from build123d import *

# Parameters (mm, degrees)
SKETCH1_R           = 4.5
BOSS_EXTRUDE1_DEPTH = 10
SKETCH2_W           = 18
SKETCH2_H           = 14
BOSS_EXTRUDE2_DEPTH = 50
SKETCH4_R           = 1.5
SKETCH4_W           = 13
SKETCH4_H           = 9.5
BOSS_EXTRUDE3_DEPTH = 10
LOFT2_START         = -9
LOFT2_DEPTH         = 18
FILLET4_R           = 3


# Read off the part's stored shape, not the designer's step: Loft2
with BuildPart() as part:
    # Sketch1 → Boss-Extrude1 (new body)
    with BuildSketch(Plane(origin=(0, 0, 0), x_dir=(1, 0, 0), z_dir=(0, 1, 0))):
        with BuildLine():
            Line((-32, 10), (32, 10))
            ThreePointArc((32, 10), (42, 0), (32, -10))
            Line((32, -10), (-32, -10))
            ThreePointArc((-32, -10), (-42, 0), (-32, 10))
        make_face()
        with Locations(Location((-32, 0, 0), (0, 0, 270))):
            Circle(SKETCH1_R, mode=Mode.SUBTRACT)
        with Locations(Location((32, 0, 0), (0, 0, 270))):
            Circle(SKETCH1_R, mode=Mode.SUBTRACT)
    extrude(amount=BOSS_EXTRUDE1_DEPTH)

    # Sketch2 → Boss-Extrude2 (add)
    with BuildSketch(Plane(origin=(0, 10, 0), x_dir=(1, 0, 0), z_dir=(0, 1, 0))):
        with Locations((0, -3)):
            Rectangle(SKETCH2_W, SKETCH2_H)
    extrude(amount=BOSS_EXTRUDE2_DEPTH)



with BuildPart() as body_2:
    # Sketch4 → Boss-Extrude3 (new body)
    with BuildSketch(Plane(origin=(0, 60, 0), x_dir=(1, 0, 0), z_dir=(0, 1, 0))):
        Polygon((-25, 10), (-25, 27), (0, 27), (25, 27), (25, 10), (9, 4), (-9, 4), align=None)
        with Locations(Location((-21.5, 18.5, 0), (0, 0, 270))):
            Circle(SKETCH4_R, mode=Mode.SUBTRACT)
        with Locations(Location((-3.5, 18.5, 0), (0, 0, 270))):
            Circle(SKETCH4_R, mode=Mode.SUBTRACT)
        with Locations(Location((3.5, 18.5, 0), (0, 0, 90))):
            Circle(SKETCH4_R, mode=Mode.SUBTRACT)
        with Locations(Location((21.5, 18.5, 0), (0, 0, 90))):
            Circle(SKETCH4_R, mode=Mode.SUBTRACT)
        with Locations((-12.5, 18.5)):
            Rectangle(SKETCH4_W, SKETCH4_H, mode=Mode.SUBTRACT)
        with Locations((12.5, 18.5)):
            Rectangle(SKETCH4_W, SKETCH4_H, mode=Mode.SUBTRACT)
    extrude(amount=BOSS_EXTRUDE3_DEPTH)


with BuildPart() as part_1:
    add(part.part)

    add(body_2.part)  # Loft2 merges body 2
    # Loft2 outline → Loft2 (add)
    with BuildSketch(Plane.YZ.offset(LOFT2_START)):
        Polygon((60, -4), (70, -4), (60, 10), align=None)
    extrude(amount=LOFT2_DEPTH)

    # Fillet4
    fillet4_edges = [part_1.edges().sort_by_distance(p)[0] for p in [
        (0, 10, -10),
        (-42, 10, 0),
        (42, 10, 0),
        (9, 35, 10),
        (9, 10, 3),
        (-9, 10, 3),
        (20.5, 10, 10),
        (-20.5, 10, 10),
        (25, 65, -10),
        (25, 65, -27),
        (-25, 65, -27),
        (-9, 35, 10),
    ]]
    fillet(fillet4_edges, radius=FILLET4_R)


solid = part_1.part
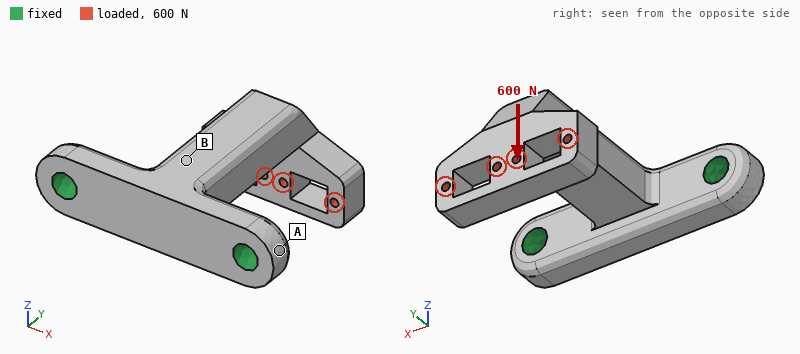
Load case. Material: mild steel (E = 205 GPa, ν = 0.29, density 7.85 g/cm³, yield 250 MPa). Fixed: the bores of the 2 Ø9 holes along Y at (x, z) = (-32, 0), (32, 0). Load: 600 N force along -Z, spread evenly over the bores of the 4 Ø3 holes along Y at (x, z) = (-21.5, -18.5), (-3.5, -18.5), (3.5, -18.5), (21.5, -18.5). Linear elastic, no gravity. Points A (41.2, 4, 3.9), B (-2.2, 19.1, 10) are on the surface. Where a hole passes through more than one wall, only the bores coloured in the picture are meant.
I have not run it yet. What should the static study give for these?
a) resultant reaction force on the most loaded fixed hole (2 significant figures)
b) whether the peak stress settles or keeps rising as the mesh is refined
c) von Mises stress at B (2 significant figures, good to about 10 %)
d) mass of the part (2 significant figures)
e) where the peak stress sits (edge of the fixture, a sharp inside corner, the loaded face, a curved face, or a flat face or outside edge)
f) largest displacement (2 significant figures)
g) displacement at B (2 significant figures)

300 N
keeps rising
48 MPa
280 g
a sharp inside corner
0.14 mm
0.023 mm
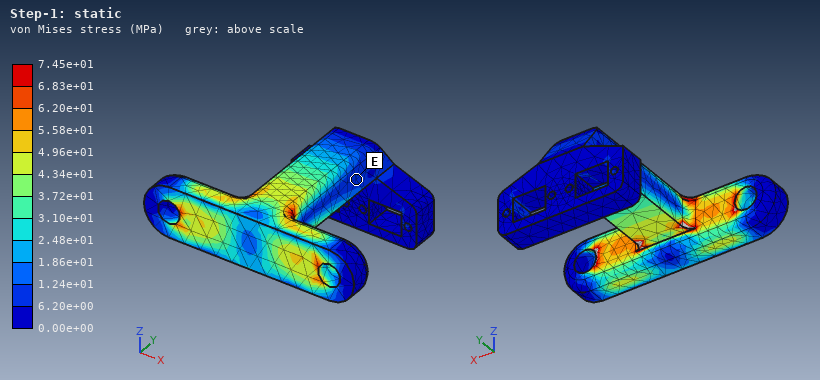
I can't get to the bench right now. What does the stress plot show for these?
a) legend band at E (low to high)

6.20e+00 to 1.24e+01 MPa
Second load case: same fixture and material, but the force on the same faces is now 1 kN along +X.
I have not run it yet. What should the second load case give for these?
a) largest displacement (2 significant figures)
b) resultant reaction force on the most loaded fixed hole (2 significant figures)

0.15 mm
1.5 kN
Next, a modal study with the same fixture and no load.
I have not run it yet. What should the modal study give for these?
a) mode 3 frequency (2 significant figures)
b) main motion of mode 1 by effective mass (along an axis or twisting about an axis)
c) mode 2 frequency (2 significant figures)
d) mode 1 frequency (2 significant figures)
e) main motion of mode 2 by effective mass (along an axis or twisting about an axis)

3600 Hz
along Z
1700 Hz
1100 Hz
along X
